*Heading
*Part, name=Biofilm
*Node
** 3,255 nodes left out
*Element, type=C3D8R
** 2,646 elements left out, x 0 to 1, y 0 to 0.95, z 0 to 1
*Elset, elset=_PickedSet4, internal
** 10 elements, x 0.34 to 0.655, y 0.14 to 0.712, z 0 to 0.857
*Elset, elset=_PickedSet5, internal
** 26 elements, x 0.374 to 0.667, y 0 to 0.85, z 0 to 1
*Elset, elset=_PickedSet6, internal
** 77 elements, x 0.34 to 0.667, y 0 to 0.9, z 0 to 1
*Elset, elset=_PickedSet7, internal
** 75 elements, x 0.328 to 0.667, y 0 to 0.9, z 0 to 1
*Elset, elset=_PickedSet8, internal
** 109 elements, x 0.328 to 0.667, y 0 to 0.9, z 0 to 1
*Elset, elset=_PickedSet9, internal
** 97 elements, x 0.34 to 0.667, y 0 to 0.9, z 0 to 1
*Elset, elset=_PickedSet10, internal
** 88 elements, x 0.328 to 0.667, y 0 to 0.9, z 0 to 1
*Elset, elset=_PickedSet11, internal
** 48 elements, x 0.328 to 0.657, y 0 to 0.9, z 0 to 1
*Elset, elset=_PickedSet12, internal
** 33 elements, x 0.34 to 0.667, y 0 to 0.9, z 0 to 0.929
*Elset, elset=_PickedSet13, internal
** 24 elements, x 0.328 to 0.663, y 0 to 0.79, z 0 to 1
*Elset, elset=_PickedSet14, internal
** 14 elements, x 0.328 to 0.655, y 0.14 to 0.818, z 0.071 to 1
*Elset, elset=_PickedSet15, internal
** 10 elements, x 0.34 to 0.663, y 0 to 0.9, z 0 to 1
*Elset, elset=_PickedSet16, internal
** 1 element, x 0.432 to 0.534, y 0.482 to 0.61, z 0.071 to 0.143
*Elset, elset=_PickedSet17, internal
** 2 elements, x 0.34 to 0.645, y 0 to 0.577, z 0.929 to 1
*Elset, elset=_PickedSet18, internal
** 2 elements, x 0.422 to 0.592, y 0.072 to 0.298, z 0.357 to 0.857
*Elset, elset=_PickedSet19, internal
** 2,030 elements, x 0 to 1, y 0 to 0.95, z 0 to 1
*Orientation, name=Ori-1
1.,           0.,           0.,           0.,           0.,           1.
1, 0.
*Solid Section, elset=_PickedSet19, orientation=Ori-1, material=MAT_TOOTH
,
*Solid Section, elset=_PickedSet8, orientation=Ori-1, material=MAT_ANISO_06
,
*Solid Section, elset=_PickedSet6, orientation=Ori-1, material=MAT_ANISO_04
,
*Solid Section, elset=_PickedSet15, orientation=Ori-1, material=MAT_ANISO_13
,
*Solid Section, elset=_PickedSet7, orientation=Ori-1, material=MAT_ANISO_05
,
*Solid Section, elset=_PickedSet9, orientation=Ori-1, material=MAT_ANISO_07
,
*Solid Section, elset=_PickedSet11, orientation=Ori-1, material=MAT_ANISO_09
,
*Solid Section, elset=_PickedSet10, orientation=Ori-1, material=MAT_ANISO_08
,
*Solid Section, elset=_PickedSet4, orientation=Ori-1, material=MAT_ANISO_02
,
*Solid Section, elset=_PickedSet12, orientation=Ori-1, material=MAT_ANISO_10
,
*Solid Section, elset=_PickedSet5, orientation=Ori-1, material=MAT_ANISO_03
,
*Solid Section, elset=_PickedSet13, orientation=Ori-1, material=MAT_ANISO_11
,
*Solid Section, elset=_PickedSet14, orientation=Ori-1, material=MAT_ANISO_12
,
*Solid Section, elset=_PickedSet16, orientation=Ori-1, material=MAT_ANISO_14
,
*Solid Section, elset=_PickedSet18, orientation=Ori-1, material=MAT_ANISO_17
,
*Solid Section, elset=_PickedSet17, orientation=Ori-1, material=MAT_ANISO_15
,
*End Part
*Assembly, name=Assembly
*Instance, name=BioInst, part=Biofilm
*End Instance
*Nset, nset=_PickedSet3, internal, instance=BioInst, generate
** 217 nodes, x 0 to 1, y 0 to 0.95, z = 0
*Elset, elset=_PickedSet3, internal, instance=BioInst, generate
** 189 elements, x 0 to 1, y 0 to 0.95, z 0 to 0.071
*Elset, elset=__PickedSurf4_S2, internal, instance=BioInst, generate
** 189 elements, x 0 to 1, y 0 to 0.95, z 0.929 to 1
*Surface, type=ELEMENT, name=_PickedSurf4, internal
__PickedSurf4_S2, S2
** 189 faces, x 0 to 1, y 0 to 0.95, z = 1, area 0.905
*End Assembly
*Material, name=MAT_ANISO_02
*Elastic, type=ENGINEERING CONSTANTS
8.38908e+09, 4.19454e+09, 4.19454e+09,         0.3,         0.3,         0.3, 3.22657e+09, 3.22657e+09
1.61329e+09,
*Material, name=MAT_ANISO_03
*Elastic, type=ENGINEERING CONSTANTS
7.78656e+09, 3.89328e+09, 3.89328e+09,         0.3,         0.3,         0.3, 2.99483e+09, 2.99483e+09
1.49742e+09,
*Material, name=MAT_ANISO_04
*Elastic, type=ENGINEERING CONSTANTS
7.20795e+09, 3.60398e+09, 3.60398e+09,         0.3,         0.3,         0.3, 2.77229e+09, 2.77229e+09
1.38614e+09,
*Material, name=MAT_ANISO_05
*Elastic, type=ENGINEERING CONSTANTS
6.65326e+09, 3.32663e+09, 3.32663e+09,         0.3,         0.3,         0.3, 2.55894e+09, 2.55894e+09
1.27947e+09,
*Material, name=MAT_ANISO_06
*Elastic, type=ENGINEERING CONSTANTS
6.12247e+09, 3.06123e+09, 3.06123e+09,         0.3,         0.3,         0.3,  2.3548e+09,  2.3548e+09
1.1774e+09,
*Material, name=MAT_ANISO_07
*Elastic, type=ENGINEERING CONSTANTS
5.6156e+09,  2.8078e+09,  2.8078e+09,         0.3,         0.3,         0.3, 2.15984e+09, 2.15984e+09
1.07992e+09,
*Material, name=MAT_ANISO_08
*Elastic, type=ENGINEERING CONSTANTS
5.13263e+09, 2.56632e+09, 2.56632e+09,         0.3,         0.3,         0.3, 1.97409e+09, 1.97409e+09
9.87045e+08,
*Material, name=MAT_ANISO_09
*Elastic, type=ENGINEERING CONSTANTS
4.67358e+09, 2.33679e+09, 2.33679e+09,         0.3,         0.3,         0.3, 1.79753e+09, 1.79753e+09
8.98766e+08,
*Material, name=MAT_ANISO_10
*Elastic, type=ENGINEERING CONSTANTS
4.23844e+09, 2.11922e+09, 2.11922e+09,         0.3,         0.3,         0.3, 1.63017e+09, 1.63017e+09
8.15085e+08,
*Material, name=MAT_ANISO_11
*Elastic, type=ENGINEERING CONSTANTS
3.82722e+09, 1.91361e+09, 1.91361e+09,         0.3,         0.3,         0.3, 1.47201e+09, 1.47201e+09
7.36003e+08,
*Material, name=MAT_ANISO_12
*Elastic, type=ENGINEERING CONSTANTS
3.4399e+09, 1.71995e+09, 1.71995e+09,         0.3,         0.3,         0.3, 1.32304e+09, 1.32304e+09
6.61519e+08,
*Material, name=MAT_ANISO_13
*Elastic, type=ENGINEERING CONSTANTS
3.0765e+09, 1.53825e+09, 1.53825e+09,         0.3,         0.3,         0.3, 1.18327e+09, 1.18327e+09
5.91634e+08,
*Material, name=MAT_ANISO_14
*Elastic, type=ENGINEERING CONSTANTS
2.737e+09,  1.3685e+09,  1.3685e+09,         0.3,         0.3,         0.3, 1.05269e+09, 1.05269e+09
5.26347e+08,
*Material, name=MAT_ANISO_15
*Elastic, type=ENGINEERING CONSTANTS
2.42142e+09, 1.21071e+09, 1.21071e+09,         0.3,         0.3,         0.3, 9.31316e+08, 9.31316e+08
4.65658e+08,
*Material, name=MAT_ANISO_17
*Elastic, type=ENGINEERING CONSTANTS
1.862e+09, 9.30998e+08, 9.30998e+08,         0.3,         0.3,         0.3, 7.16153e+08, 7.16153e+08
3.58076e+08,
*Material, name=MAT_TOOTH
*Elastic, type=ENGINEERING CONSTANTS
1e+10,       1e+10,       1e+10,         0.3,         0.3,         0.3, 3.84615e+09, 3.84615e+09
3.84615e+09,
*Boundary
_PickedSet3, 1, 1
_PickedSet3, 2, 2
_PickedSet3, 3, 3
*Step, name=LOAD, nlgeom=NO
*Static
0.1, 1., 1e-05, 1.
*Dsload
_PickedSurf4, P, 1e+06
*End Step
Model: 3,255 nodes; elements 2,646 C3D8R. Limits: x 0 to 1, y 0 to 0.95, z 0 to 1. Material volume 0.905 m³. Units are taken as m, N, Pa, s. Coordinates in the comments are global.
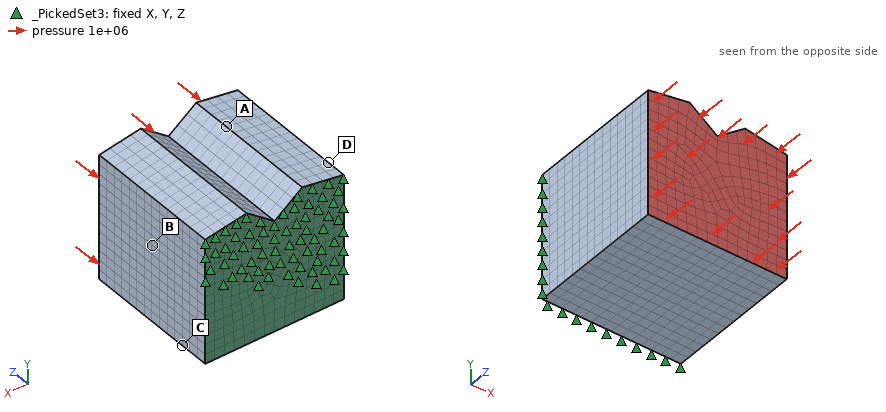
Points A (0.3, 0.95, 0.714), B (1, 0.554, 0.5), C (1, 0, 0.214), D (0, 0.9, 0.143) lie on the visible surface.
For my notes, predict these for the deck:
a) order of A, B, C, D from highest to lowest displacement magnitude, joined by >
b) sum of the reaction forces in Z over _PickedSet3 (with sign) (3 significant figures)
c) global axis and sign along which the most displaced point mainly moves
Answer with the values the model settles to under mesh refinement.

A > B > C > D
9.05e+05 N
-Z
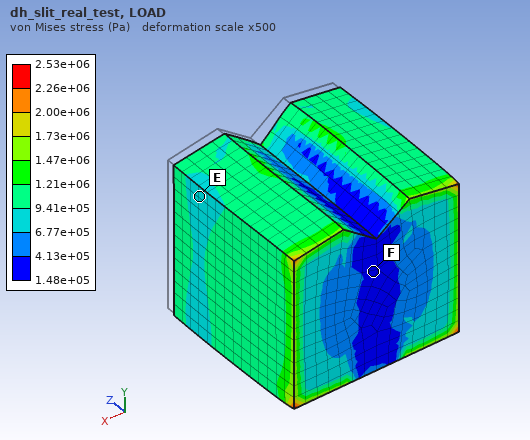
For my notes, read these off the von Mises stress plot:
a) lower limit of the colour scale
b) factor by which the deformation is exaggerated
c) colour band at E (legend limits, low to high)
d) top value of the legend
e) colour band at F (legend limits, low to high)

1.48e+05 Pa
500
6.77e+05 to 9.41e+05 Pa
2.53e+06 Pa
1.48e+05 to 4.13e+05 Pa
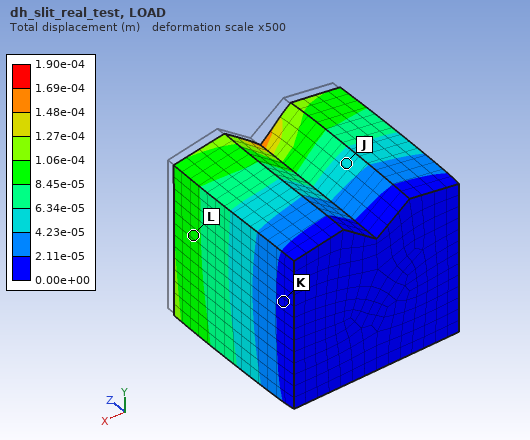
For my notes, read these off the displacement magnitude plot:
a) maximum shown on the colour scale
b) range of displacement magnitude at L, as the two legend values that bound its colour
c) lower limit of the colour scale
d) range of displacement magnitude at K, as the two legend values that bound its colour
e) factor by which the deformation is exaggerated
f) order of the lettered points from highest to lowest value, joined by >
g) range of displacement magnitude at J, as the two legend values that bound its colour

1.90e-04 m
8.45e-05 to 1.06e-04 m
0.00e+00 m
0.00e+00 to 2.11e-05 m
500
L > J > K
4.23e-05 to 6.34e-05 m
